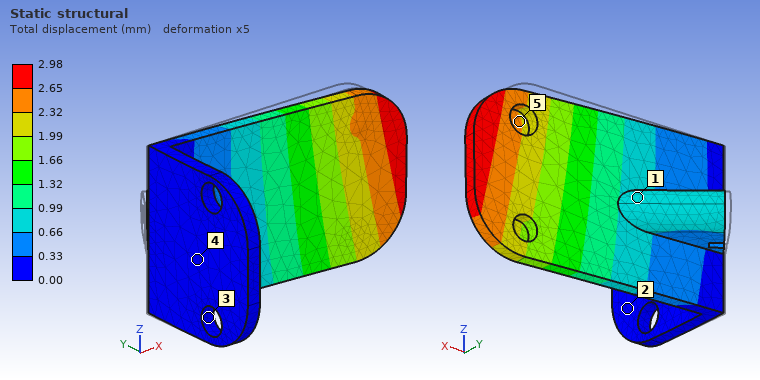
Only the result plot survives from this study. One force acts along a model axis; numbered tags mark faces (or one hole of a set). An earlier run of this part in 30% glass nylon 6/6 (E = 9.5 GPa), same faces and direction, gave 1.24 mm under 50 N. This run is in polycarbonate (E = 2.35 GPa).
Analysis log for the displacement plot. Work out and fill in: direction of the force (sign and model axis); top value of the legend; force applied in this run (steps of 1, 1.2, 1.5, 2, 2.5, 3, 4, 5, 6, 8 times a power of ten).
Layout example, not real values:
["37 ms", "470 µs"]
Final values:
["-Y", "2.98 mm", "30 N"]
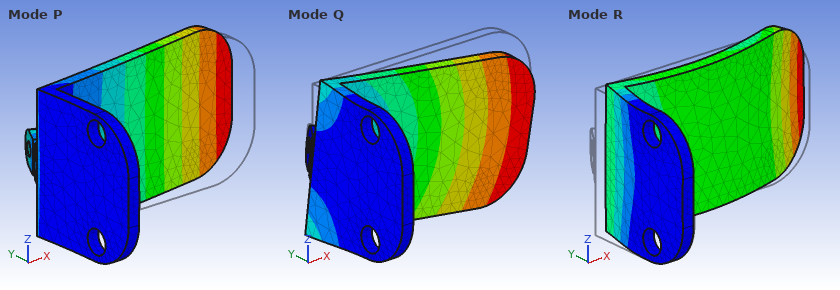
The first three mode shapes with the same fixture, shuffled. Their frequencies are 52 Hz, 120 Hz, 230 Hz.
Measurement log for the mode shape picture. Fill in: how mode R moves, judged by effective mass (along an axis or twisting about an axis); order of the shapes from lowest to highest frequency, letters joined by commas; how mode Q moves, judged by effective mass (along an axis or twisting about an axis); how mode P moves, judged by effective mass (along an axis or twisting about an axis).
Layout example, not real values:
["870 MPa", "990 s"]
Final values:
["along X", "P, Q, R", "along Z", "along Y"]
